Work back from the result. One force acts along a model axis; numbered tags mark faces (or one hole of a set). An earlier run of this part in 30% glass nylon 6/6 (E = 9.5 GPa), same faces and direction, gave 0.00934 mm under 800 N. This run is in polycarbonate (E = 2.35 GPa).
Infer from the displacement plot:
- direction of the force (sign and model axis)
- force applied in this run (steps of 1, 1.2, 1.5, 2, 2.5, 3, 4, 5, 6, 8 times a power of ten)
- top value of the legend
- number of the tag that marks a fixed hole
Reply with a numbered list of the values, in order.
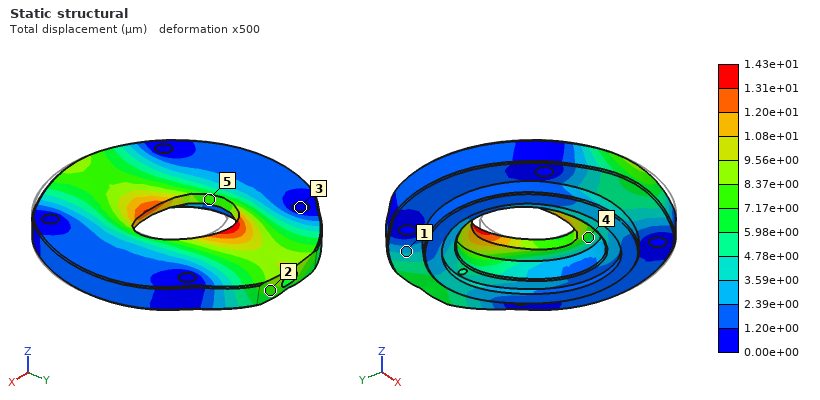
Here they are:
1. +Y
2. 300 N
3. 1.43e+01 µm
4. 3
